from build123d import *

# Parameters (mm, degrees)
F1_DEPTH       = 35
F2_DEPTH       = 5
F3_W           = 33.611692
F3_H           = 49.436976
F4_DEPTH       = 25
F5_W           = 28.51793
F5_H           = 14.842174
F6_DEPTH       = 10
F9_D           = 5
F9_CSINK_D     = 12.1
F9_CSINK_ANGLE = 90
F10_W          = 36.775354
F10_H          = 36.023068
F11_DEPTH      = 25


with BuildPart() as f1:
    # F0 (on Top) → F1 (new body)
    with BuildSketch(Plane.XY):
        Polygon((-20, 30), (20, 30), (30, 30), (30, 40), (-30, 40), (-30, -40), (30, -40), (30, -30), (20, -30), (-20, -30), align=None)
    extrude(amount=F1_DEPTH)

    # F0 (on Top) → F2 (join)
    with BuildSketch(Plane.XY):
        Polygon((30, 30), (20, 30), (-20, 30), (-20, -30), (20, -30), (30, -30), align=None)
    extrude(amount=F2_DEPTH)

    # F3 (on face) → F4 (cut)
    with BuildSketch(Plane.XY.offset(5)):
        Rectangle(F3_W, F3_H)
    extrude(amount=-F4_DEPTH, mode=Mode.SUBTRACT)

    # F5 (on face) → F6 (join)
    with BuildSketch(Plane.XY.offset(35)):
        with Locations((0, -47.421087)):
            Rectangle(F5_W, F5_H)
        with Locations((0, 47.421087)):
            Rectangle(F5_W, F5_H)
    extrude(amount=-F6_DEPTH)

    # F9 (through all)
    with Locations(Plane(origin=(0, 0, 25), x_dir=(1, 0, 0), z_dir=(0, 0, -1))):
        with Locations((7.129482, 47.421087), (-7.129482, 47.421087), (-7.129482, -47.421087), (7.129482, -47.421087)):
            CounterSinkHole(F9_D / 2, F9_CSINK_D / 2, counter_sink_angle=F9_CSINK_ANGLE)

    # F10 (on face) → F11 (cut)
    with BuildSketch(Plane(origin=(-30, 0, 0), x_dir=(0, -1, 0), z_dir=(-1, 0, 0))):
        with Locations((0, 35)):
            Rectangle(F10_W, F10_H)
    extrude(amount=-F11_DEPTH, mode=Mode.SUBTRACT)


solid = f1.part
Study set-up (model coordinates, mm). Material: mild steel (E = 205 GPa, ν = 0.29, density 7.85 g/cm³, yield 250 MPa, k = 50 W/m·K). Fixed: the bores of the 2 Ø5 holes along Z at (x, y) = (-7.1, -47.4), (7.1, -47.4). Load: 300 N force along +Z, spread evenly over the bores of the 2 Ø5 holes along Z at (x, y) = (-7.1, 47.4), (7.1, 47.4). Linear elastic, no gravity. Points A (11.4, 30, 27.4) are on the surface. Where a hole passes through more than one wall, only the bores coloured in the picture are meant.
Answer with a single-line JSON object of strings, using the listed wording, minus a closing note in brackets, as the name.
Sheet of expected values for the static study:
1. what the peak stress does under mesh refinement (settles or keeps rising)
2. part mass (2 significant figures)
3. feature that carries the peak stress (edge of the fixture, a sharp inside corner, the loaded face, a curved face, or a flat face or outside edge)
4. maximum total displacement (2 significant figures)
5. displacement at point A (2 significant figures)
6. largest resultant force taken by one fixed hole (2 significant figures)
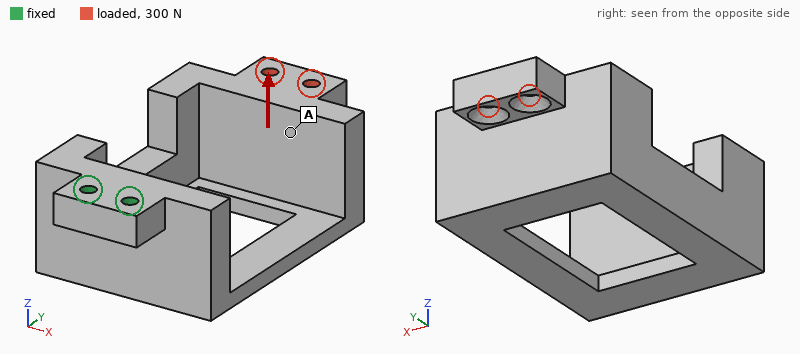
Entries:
{"what the peak stress does under mesh refinement": "keeps rising", "part mass": "550 g", "feature that carries the peak stress": "edge of the fixture", "maximum total displacement": "0.21 mm", "displacement at point A": "0.15 mm", "largest resultant force taken by one fixed hole": "260 N"}
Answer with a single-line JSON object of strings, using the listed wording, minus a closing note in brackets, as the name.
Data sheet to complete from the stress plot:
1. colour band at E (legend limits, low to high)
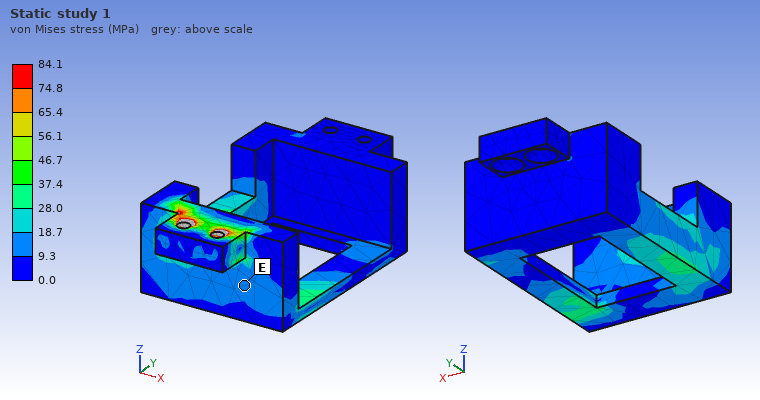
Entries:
{"colour band at E": "9.3 to 18.7 MPa"}
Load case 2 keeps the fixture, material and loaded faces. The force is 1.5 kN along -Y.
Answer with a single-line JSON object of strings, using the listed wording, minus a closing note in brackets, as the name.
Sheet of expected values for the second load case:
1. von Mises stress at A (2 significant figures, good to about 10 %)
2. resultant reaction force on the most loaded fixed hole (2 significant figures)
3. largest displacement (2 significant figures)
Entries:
{"von Mises stress at A": "24 MPa", "resultant reaction force on the most loaded fixed hole": "840 N", "largest displacement": "0.24 mm"}
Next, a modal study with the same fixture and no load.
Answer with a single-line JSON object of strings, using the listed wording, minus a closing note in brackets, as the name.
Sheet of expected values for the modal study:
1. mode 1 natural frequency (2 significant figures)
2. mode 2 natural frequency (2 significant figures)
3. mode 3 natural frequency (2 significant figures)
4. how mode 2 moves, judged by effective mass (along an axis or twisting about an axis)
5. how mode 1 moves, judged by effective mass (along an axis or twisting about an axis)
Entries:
{"mode 1 natural frequency": "470 Hz", "mode 2 natural frequency": "730 Hz", "mode 3 natural frequency": "1500 Hz", "how mode 2 moves, judged by effective mass": "along X", "how mode 1 moves, judged by effective mass": "along Z"}
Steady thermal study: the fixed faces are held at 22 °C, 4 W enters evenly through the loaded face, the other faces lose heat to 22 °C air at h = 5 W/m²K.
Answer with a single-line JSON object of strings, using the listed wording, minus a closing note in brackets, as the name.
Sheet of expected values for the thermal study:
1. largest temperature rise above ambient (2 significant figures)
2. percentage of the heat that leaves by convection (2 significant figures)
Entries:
{"largest temperature rise above ambient": "26 K", "percentage of the heat that leaves by convection": "31 %"}
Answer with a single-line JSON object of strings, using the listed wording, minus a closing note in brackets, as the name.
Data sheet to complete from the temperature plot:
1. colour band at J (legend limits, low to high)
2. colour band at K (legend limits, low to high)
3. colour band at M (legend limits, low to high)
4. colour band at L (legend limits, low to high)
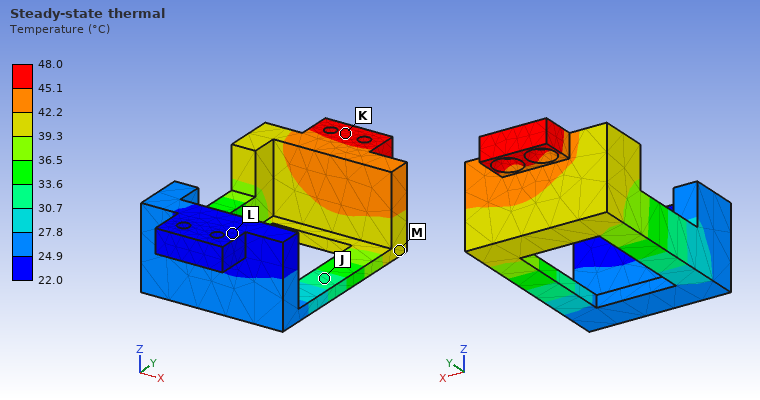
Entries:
{"colour band at J": "30.7 to 33.6 °C", "colour band at K": "45.1 to 48.0 °C", "colour band at M": "39.3 to 42.2 °C", "colour band at L": "22.0 to 24.9 °C"}
